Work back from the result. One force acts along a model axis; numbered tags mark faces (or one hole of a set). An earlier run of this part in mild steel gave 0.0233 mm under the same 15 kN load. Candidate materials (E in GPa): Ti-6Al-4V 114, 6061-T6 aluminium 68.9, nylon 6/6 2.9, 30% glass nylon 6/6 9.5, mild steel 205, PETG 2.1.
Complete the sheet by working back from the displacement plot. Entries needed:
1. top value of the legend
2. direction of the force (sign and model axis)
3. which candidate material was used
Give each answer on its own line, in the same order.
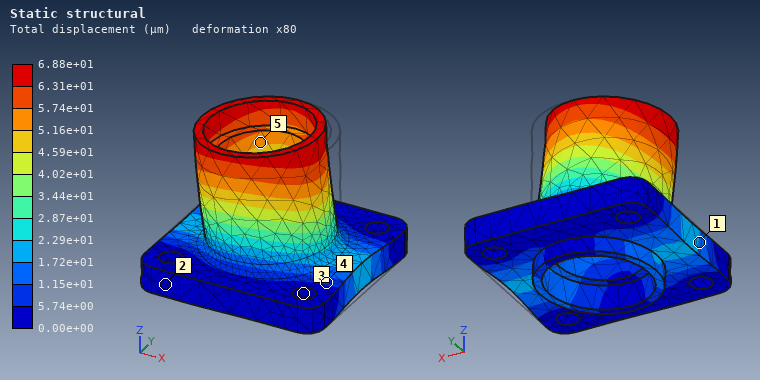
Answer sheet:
6.88e+01 µm
-X
6061-T6 aluminium
